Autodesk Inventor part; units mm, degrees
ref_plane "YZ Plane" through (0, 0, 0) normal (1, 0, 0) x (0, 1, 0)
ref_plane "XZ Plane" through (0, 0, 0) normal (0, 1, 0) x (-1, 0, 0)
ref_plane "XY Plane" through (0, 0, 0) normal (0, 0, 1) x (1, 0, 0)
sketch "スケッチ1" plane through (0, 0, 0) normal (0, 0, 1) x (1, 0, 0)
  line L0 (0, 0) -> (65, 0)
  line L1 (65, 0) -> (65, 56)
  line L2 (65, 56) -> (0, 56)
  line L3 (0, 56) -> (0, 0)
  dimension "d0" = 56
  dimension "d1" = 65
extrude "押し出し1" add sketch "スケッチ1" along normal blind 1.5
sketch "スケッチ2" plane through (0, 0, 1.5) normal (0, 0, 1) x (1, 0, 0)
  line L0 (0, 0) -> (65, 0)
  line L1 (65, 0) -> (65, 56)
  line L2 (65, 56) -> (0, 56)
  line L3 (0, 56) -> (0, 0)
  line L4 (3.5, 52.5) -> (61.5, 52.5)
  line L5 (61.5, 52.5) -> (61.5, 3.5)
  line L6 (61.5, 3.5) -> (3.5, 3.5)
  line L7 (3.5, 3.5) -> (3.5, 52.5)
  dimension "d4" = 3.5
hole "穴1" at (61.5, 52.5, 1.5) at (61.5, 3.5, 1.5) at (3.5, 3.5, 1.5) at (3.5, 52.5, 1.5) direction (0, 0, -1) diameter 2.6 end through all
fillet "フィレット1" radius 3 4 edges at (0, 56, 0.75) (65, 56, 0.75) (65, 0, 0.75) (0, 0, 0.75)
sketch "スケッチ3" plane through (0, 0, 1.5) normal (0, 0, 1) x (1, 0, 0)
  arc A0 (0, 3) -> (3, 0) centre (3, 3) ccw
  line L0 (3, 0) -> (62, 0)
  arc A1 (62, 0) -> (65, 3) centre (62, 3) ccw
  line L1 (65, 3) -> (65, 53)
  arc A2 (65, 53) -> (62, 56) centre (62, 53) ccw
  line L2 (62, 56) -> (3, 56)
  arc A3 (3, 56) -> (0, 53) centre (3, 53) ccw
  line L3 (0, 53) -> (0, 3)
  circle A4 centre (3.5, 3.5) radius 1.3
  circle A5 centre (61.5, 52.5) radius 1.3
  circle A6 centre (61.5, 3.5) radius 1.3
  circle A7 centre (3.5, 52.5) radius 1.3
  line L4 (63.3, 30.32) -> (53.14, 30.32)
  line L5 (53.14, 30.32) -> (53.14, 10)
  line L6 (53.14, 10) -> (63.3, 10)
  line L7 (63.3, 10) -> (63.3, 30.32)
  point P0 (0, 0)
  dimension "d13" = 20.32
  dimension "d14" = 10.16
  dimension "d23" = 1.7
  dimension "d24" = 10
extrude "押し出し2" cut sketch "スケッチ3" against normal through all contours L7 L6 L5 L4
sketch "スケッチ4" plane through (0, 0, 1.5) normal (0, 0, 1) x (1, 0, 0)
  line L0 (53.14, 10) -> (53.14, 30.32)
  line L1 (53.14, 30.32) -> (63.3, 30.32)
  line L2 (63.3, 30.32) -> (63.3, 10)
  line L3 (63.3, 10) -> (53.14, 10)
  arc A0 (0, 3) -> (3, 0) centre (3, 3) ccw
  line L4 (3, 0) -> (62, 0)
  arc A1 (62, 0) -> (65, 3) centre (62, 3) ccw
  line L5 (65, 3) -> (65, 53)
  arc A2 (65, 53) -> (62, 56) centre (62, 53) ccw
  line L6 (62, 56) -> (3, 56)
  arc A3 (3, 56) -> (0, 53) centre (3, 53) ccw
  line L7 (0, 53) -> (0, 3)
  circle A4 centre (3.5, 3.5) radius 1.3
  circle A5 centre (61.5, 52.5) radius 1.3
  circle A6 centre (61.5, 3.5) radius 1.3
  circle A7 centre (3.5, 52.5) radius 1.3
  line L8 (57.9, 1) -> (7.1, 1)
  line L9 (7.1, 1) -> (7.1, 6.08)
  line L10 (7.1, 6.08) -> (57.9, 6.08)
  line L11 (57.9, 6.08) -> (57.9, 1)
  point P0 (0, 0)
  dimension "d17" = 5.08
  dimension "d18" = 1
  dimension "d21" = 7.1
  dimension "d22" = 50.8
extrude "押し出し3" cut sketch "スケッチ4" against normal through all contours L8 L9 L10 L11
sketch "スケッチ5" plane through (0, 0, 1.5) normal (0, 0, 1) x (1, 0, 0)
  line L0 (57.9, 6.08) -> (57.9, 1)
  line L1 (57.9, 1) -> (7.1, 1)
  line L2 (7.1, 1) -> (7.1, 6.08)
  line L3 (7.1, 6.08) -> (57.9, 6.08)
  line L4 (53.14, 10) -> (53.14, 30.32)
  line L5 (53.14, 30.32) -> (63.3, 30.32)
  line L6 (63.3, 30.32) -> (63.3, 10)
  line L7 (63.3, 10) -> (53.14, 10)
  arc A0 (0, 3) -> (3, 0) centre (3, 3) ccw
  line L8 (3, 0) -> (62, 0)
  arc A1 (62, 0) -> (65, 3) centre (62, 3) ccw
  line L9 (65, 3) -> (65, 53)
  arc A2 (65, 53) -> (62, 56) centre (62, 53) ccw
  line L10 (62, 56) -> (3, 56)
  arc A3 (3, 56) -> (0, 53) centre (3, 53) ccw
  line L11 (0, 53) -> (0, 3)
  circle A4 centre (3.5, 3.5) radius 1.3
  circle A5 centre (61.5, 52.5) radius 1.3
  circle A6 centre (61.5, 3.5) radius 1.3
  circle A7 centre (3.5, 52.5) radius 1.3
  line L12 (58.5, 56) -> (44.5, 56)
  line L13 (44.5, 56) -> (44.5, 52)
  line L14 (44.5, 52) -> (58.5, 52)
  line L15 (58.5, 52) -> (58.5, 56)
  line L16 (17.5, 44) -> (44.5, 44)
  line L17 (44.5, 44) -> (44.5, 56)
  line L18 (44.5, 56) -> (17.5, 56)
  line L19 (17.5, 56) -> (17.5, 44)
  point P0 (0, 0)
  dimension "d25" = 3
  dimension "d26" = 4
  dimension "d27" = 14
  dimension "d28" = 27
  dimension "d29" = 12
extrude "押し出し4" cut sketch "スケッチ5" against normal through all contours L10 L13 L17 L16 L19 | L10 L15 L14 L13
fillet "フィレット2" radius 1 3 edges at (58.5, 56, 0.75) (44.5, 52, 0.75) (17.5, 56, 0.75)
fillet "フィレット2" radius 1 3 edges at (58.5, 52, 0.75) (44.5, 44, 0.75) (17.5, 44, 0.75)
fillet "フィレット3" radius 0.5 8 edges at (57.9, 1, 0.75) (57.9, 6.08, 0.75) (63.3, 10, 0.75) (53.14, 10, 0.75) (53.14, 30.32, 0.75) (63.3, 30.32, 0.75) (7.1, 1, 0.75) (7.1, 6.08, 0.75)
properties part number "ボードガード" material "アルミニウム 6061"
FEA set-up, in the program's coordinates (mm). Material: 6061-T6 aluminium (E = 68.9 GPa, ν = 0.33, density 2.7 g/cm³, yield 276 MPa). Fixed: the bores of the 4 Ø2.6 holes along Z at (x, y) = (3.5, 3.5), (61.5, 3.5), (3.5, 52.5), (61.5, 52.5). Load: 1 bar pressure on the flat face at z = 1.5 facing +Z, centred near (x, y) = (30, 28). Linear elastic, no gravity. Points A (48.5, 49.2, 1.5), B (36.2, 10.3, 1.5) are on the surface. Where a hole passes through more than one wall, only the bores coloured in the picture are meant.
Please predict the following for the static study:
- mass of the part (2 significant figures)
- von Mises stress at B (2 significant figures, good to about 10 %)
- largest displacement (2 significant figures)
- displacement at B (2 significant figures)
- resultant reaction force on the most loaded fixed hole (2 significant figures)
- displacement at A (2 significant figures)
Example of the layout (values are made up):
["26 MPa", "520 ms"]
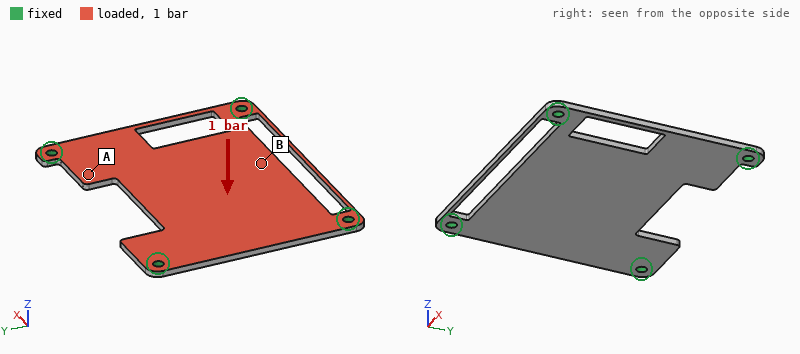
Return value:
["11 g", "55 MPa", "0.35 mm", "0.31 mm", "76 N", "0.14 mm"]
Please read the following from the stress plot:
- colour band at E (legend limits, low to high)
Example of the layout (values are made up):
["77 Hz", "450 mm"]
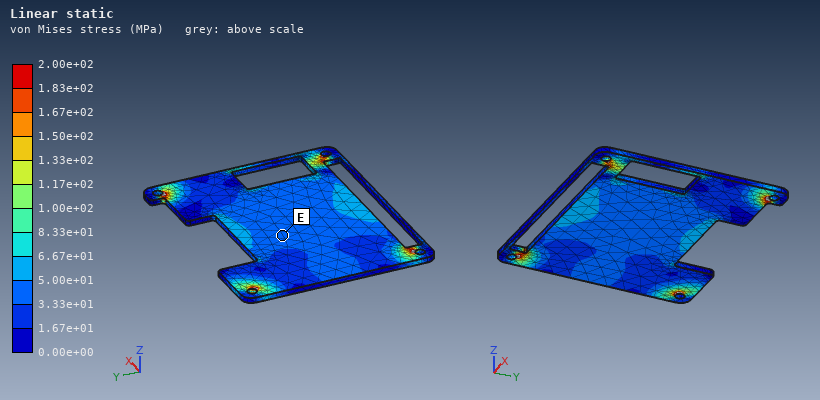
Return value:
["3.33e+01 to 5.00e+01 MPa"]
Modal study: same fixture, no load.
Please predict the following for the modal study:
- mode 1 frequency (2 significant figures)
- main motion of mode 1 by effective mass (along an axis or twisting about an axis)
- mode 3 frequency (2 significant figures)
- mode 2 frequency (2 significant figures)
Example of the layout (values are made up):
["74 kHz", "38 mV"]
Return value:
["1500 Hz", "along Z", "2700 Hz", "2000 Hz"]
